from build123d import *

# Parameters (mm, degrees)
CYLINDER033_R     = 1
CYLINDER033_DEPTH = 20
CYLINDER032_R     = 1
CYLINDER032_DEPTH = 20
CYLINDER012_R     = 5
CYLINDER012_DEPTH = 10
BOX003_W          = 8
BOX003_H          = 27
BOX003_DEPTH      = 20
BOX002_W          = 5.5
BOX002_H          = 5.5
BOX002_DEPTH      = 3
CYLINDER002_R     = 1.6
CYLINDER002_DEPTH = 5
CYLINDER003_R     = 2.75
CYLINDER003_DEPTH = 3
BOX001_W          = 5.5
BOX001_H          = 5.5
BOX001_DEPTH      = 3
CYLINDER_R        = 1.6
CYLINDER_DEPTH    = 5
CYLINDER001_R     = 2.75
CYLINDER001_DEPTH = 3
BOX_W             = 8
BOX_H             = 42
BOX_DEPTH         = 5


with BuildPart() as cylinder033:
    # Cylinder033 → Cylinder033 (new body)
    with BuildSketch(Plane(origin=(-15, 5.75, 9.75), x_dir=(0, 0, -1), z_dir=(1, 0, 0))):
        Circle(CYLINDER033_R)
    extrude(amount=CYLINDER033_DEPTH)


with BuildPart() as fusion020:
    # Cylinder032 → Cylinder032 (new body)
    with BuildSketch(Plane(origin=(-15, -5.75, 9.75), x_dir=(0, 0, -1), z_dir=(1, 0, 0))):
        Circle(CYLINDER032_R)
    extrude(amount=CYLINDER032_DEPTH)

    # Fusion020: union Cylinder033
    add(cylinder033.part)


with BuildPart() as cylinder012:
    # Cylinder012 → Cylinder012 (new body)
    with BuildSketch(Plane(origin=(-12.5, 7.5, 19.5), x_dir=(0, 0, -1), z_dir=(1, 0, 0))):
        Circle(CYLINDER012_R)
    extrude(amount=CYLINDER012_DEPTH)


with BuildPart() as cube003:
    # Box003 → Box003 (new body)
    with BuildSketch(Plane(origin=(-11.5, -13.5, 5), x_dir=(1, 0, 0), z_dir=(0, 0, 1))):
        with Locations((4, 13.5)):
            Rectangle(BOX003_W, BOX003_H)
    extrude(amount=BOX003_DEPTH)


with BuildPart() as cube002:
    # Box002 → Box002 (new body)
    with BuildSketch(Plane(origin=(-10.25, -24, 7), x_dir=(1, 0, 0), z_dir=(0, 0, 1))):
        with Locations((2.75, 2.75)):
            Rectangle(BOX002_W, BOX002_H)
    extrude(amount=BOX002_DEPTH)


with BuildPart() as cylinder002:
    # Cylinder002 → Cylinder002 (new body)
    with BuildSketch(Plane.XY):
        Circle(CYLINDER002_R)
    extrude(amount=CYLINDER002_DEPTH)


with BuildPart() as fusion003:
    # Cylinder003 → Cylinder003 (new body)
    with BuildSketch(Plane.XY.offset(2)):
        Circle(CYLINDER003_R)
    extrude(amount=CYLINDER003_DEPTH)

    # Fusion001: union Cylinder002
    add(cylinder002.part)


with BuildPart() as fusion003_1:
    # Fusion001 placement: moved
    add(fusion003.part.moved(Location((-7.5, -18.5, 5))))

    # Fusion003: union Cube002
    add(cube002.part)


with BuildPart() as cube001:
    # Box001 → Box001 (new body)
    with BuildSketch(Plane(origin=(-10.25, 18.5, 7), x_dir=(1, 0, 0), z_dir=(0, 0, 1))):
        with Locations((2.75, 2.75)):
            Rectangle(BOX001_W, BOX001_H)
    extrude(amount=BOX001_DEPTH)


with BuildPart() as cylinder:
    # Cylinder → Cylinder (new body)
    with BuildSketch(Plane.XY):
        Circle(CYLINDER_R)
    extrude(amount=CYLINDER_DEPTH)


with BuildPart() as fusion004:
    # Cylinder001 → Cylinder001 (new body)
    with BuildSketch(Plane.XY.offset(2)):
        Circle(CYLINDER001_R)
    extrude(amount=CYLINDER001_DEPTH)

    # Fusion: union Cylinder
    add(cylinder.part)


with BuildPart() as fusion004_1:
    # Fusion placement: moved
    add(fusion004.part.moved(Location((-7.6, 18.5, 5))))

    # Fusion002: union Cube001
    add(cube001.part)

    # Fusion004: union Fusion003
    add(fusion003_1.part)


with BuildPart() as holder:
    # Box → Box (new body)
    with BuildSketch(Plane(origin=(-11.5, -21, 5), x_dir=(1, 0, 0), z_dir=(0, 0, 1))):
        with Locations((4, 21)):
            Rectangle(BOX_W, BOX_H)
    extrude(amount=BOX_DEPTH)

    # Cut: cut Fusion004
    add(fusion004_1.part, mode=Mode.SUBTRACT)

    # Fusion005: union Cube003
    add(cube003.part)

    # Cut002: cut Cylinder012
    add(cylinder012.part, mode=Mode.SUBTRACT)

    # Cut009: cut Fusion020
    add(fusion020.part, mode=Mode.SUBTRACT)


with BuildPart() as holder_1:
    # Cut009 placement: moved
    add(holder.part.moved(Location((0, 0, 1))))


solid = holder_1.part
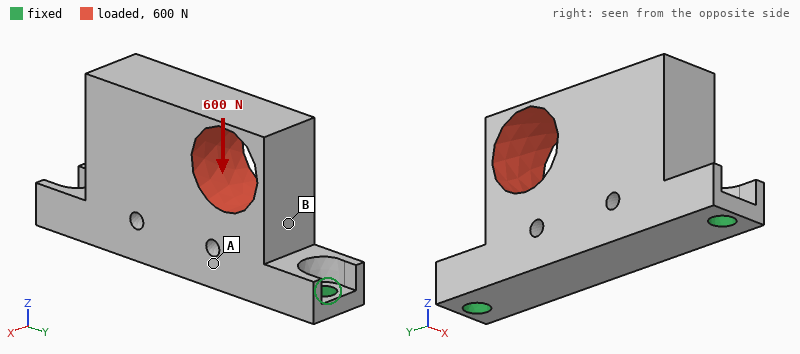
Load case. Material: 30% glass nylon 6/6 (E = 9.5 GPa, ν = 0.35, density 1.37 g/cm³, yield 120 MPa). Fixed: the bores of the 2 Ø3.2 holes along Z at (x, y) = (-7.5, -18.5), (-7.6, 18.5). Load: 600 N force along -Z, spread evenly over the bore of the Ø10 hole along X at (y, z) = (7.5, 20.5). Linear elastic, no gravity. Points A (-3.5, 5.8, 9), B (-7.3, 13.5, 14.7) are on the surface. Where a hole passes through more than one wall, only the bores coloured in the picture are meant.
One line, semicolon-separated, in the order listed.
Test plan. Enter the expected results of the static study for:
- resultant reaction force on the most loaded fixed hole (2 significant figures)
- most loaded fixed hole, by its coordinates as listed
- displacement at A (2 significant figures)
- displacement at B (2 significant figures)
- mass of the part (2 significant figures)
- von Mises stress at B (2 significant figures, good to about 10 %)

510 N; (-7.6, 18.5); 0.061 mm; 0.062 mm; 5.6 g; 28 MPa
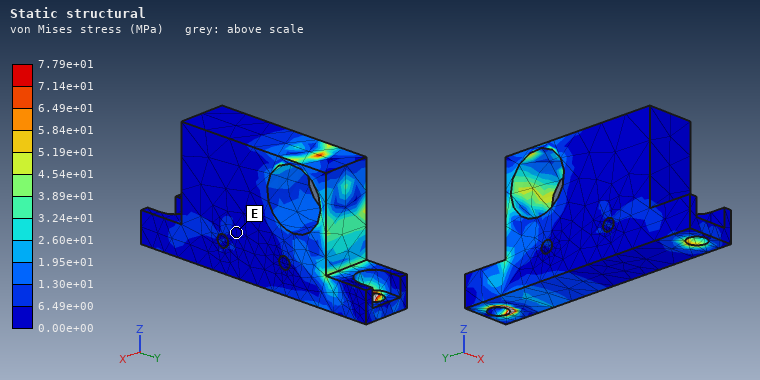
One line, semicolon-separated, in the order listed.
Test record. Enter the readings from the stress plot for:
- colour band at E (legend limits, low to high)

0.00e+00 to 6.49e+00 MPa
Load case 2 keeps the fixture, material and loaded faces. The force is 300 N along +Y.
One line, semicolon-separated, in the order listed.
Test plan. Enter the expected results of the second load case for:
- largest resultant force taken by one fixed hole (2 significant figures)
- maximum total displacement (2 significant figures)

200 N; 50 µm
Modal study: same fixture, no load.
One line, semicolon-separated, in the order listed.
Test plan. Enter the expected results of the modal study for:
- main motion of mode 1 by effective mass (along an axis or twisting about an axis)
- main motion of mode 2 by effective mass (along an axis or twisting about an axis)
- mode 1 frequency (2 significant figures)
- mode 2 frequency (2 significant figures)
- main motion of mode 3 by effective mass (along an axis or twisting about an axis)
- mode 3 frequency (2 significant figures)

along X; along Z; 2200 Hz; 7900 Hz; along X; 9500 Hz
